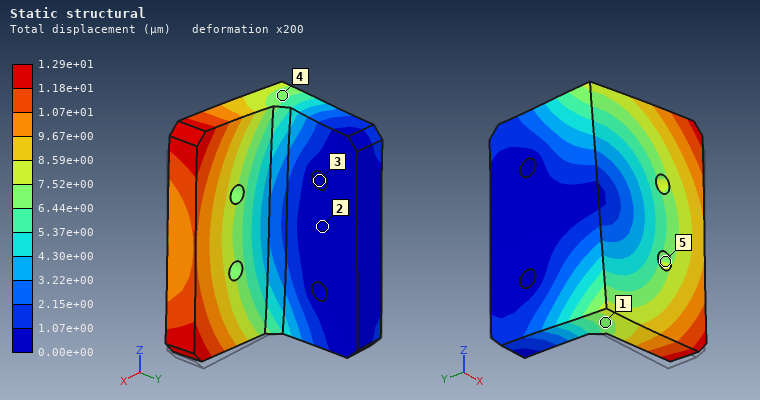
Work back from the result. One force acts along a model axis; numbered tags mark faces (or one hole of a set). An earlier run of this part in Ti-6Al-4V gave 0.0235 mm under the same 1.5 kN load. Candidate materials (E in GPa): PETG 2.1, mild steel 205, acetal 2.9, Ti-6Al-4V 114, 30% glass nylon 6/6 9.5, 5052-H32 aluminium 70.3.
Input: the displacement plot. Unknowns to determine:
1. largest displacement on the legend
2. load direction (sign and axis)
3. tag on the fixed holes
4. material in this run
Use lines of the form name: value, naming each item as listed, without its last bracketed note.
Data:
largest displacement on the legend: 1.29e+01 µm
load direction: +Z
tag on the fixed holes: 3
material in this run: mild steel
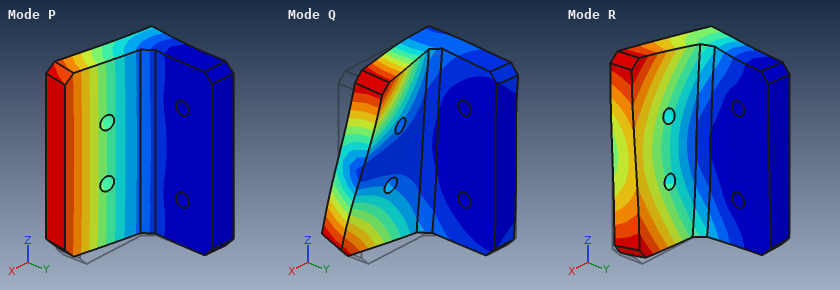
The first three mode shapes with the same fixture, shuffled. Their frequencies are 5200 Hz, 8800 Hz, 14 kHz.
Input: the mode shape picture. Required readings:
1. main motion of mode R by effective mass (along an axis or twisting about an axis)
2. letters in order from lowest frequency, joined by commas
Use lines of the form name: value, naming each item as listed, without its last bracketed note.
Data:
main motion of mode R by effective mass: along Z
letters in order from lowest frequency, joined by commas: P, R, Q
